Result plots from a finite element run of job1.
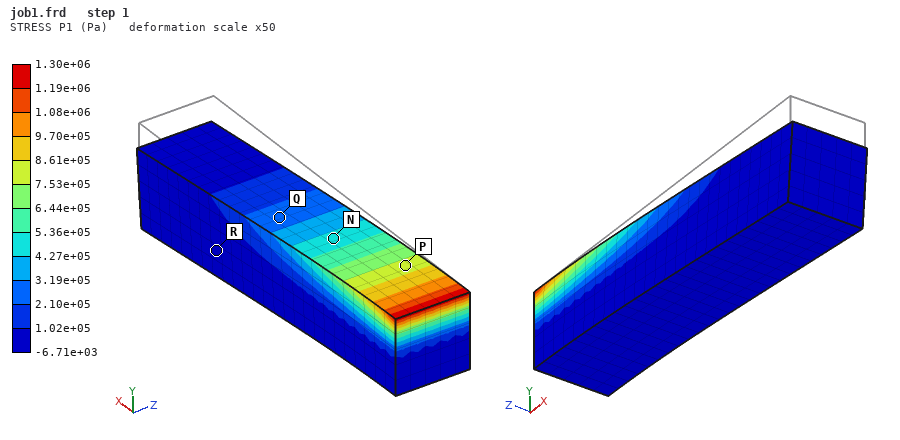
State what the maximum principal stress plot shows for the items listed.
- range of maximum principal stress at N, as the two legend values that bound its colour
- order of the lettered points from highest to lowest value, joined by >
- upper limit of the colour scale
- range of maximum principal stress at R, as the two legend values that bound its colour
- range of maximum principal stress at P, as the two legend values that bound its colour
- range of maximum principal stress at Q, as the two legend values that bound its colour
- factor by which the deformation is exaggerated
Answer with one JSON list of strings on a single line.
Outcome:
["4.27e+05 to 5.36e+05 Pa", "P > N > Q > R", "1.30e+06 Pa", "-6.71e+03 to 1.02e+05 Pa", "7.53e+05 to 8.61e+05 Pa", "2.10e+05 to 3.19e+05 Pa", "50"]
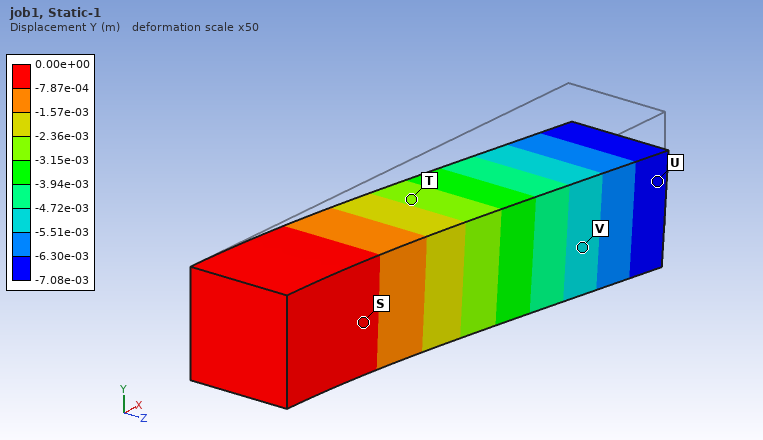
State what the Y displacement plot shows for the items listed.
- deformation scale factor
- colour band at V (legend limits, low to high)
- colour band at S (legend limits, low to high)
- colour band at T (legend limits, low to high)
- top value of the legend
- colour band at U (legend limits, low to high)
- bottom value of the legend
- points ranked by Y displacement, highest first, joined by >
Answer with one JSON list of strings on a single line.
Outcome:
["50", "-5.51e-03 to -4.72e-03 m", "-7.87e-04 to 0.00e+00 m", "-3.15e-03 to -2.36e-03 m", "0.00e+00 m", "-7.08e-03 to -6.30e-03 m", "-7.08e-03 m", "S > T > V > U"]
